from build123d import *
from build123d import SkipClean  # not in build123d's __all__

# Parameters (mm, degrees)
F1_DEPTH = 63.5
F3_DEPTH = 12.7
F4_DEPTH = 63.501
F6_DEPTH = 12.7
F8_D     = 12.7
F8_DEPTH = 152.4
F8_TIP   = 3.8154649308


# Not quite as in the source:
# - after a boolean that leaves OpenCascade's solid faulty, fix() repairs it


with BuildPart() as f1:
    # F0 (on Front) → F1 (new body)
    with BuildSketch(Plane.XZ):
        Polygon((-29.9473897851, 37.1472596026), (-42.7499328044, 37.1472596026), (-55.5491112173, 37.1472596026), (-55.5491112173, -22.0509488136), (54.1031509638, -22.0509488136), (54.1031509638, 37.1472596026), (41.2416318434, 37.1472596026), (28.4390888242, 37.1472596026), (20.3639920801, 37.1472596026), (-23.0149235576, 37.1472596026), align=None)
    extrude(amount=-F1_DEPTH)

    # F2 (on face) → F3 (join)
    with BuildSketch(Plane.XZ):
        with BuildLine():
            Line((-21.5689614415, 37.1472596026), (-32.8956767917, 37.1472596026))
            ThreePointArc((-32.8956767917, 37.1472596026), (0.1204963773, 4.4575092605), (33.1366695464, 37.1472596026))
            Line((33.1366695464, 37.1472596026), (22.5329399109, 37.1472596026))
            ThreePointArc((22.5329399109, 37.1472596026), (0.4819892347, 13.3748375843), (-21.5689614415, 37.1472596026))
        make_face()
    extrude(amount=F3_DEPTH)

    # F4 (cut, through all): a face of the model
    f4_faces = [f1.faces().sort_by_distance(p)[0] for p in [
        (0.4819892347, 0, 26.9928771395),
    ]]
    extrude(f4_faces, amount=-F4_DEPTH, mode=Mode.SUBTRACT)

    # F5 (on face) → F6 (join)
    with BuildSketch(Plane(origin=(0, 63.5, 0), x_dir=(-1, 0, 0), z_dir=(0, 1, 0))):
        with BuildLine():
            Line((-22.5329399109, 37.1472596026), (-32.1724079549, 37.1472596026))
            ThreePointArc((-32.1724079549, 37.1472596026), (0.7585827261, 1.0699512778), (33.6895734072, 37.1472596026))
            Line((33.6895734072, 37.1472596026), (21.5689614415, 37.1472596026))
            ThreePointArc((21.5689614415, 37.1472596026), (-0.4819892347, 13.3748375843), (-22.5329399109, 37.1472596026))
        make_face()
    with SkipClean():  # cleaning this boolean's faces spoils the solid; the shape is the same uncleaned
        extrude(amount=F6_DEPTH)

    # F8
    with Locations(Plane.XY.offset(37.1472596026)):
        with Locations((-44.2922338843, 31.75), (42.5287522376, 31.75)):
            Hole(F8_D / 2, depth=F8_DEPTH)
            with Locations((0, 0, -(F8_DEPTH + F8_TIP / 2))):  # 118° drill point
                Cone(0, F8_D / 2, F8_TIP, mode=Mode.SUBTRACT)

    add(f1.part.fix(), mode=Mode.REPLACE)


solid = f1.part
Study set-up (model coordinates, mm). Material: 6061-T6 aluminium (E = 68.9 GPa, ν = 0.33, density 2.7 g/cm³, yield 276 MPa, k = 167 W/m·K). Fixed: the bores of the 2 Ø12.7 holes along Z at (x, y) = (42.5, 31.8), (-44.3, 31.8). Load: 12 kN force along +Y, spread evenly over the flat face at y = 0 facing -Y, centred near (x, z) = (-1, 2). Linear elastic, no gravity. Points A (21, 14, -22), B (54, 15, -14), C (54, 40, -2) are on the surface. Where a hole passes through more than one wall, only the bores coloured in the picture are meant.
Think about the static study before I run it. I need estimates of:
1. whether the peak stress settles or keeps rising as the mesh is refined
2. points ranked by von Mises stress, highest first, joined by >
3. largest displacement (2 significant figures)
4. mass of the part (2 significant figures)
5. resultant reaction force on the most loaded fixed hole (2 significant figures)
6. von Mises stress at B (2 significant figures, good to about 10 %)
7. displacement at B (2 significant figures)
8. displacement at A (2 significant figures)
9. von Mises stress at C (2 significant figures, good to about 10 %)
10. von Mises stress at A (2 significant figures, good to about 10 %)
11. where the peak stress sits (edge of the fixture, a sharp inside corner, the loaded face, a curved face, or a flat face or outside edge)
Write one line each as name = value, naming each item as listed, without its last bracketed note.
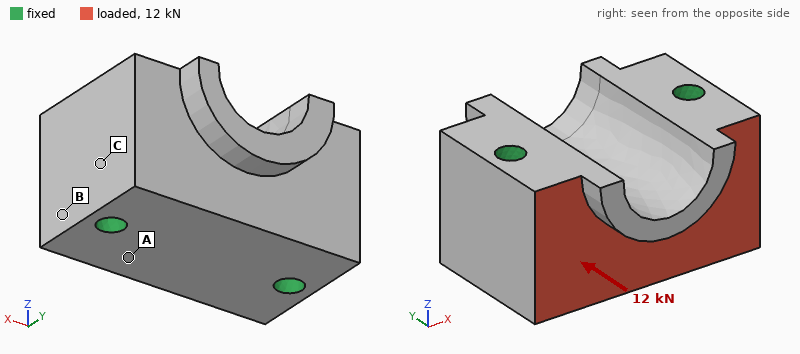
whether the peak stress settles or keeps rising as the mesh is refined = keeps rising
points ranked by von Mises stress, highest first, joined by > = A > B > C
largest displacement = 3.2 µm
mass of the part = 990 g
resultant reaction force on the most loaded fixed hole = 6.0 kN
von Mises stress at B = 2.0 MPa
displacement at B = 0.61 µm
displacement at A = 2.1 µm
von Mises stress at C = 0.86 MPa
von Mises stress at A = 2.8 MPa
where the peak stress sits = edge of the fixture
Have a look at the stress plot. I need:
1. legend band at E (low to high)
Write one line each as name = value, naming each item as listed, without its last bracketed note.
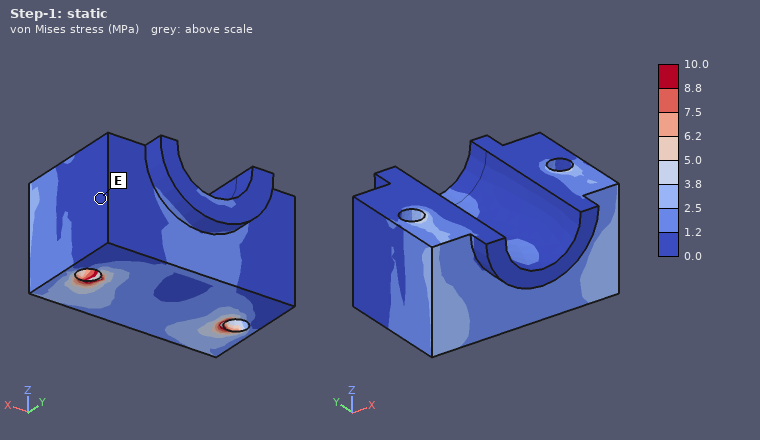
legend band at E = 0.0 to 1.2 MPa
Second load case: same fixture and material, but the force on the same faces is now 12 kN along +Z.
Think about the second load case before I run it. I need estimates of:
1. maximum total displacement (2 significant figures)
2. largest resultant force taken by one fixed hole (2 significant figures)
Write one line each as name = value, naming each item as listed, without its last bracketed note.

maximum total displacement = 8.2 µm
largest resultant force taken by one fixed hole = 6.1 kN
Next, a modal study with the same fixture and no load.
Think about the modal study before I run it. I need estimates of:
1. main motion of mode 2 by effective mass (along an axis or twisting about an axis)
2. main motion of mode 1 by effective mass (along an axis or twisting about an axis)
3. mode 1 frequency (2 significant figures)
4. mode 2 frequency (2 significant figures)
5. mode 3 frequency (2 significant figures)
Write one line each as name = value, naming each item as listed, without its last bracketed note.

main motion of mode 2 by effective mass = along Z
main motion of mode 1 by effective mass = along Y
mode 1 frequency = 13 kHz
mode 2 frequency = 13 kHz
mode 3 frequency = 14 kHz
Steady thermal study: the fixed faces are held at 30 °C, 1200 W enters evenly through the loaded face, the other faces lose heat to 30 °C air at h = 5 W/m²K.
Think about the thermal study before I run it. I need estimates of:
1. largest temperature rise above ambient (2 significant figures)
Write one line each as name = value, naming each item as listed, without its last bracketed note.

largest temperature rise above ambient = 54 K
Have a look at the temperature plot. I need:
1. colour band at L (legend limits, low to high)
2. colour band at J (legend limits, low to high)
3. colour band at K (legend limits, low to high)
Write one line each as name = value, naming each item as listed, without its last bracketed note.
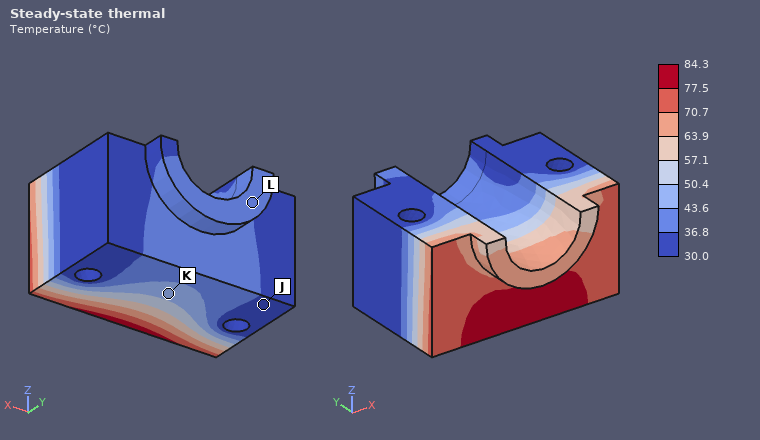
colour band at L = 36.8 to 43.6 °C
colour band at J = 30.0 to 36.8 °C
colour band at K = 43.6 to 50.4 °C
